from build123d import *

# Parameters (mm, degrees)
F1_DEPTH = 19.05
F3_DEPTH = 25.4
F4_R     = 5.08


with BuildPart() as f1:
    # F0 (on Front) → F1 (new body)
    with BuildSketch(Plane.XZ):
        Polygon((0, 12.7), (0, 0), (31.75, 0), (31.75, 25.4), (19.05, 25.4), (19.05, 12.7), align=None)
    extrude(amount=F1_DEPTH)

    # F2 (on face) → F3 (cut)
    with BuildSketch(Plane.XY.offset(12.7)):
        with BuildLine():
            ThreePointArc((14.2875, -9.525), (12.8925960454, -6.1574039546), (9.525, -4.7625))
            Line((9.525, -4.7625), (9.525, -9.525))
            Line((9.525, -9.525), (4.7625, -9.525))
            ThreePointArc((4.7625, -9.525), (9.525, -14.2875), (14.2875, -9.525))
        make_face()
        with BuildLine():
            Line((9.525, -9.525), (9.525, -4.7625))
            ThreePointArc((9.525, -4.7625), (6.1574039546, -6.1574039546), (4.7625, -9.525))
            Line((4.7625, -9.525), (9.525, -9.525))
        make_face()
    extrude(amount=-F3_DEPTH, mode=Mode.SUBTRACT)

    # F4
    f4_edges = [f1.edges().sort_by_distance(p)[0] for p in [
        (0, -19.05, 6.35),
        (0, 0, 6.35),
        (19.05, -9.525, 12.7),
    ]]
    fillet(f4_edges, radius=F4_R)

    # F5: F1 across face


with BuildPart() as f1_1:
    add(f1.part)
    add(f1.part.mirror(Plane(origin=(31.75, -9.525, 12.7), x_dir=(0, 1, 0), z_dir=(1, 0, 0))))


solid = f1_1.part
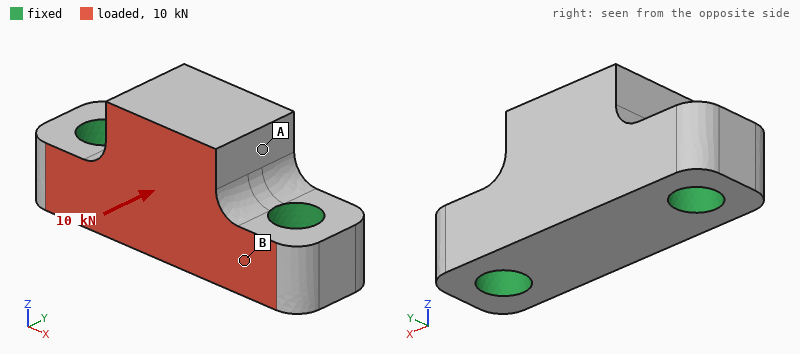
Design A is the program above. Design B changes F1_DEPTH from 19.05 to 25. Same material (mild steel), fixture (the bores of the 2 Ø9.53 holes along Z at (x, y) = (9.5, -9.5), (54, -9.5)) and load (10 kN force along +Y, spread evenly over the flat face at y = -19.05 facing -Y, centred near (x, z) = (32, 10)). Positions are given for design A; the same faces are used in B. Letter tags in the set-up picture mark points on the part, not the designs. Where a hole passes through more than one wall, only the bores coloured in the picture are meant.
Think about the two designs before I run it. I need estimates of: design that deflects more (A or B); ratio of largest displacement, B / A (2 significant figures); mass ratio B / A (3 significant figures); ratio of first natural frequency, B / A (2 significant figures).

A
0.79
1.35
0.95
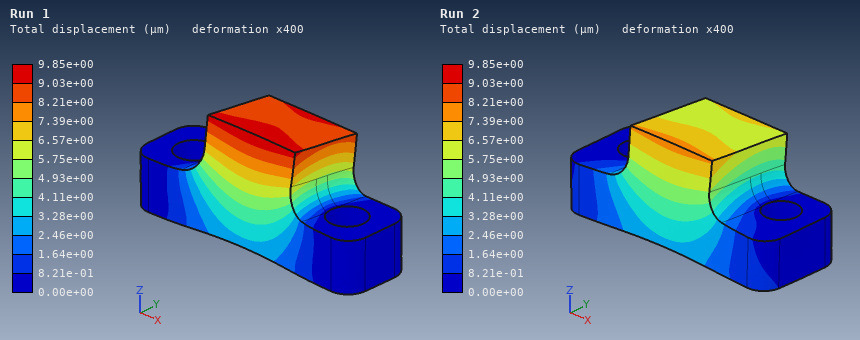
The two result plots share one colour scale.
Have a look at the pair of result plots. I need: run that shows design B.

Run 2
